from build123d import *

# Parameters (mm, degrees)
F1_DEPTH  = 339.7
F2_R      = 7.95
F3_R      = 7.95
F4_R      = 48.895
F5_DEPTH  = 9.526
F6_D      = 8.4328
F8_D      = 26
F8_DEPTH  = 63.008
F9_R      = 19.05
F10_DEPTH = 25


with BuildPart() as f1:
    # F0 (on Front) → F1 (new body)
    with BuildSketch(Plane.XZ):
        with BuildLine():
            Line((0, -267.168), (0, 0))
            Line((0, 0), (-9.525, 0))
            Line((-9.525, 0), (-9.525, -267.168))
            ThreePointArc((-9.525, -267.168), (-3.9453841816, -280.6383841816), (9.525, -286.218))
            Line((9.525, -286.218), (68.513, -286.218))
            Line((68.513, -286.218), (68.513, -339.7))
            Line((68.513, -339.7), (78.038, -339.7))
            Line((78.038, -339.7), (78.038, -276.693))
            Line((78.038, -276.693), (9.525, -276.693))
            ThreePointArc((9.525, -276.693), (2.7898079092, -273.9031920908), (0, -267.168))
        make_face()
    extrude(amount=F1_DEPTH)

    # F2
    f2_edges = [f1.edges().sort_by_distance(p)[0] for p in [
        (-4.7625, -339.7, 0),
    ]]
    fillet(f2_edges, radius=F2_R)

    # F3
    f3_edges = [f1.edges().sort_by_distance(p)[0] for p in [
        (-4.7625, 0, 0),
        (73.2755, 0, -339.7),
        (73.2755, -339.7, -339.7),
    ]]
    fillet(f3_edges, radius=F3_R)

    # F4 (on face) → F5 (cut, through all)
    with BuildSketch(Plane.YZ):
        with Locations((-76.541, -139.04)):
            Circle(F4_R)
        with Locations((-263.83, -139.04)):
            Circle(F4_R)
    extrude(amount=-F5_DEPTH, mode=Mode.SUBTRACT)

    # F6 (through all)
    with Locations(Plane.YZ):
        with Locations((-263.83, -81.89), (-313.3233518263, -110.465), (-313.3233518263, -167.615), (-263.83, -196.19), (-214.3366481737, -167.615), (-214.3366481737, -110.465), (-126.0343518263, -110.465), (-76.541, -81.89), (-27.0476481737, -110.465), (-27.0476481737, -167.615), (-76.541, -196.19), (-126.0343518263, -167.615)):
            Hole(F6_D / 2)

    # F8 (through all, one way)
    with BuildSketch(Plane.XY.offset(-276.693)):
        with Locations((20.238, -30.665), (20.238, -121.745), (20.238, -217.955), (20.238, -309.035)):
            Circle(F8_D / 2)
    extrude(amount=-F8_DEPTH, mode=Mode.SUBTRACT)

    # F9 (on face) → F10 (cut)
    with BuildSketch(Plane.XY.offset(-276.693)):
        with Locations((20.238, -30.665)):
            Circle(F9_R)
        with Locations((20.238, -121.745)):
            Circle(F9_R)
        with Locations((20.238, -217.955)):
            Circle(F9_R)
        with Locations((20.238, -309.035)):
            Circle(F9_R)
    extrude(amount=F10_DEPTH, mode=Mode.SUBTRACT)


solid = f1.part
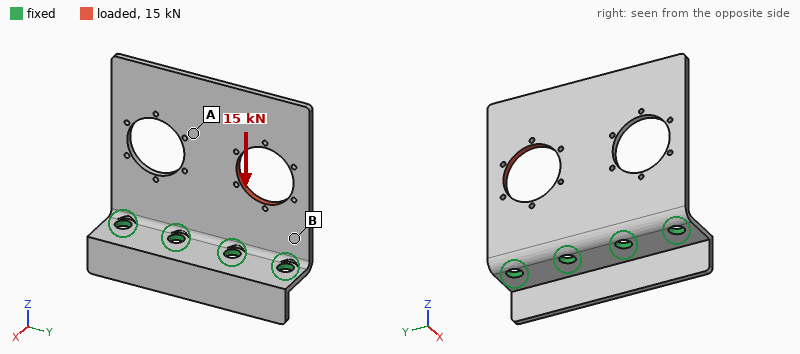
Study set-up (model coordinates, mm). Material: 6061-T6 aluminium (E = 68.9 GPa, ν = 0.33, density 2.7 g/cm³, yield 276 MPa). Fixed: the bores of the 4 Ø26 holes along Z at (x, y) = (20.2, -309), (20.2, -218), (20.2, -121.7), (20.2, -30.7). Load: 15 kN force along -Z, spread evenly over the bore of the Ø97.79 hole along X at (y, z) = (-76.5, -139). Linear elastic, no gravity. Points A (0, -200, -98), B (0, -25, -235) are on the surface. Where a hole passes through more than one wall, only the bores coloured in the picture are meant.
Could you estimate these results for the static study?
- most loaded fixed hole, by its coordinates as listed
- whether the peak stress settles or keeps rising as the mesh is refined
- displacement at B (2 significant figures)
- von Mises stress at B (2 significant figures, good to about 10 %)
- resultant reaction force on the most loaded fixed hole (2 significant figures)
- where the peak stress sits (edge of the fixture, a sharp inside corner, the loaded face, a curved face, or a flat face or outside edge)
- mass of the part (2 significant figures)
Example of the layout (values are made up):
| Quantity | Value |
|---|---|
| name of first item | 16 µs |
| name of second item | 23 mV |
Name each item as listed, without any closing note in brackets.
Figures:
| Quantity | Value |
|---|---|
| most loaded fixed hole, by its coordinates as listed | (20.2, -30.7) |
| whether the peak stress settles or keeps rising as the mesh is refined | keeps rising |
| displacement at B | 0.15 mm |
| von Mises stress at B | 17 MPa |
| resultant reaction force on the most loaded fixed hole | 8.2 kN |
| where the peak stress sits | edge of the fixture |
| mass of the part | 3.1 kg |
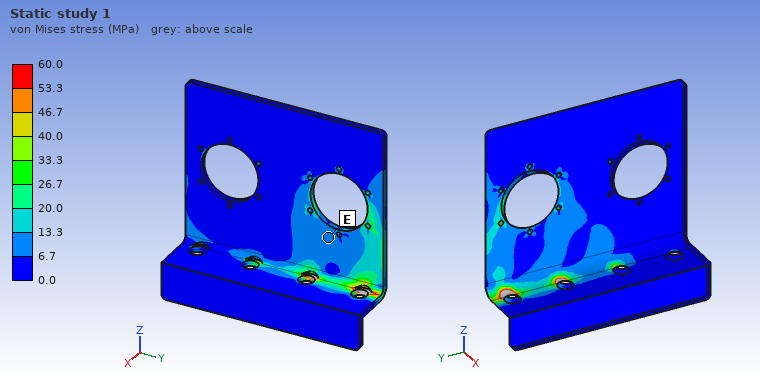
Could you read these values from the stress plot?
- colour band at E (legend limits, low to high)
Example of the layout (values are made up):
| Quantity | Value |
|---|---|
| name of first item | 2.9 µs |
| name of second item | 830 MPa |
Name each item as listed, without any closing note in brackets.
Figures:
| Quantity | Value |
|---|---|
| colour band at E | 6.7 to 13.3 MPa |
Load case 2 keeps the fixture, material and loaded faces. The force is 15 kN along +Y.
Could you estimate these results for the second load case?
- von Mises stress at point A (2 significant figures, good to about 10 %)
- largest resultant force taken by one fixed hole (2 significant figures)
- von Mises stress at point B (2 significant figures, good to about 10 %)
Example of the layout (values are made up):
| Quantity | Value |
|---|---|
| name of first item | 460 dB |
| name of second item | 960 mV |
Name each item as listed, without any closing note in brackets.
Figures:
| Quantity | Value |
|---|---|
| von Mises stress at point A | 5.3 MPa |
| largest resultant force taken by one fixed hole | 7.9 kN |
| von Mises stress at point B | 14 MPa |
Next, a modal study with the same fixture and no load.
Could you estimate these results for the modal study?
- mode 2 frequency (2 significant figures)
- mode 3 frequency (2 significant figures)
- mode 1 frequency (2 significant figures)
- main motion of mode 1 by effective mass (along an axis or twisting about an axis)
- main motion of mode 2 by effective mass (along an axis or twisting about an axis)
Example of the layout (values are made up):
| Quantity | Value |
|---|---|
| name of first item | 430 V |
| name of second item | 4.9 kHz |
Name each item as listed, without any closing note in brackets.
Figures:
| Quantity | Value |
|---|---|
| mode 2 frequency | 190 Hz |
| mode 3 frequency | 500 Hz |
| mode 1 frequency | 88 Hz |
| main motion of mode 1 by effective mass | along X |
| main motion of mode 2 by effective mass | twisting about Z |
